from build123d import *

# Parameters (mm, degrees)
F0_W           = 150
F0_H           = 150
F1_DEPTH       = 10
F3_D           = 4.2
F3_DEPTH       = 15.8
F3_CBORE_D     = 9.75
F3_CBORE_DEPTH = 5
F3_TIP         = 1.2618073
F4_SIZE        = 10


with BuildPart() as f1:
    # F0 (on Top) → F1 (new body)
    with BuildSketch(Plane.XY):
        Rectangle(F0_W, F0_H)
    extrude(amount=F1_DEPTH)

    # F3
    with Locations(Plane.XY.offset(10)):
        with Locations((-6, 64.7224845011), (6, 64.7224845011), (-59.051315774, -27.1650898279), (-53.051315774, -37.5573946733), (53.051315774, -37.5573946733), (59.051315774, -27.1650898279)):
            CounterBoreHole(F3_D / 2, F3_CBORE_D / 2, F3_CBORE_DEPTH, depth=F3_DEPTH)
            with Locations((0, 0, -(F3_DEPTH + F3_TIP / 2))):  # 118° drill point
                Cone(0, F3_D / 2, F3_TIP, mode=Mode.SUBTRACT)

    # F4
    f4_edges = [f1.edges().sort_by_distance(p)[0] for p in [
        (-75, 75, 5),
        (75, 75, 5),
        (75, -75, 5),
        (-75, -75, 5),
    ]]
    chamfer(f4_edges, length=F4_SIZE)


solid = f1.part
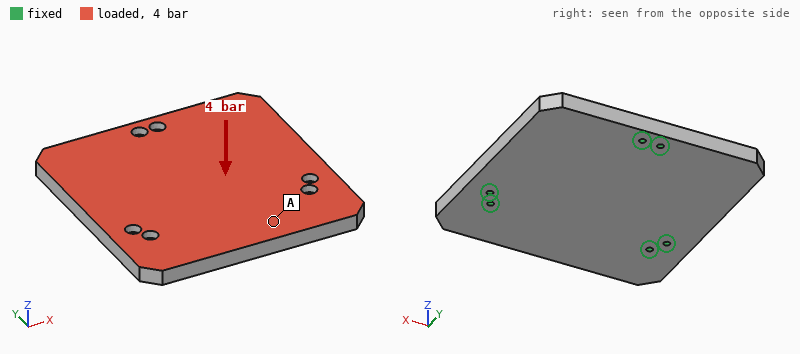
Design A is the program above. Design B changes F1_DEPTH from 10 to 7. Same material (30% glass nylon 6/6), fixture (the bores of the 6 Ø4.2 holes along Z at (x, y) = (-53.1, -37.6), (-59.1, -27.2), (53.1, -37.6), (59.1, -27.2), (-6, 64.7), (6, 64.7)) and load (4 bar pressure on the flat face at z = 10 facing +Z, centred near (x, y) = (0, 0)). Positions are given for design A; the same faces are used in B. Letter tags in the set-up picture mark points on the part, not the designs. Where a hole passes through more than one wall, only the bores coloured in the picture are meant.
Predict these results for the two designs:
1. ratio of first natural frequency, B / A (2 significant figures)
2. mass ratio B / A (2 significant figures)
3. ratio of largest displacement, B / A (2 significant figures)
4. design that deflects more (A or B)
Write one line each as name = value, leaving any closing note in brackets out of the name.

ratio of first natural frequency, B / A = 0.79
mass ratio B / A = 0.70
ratio of largest displacement, B / A = 2.6
design that deflects more = B
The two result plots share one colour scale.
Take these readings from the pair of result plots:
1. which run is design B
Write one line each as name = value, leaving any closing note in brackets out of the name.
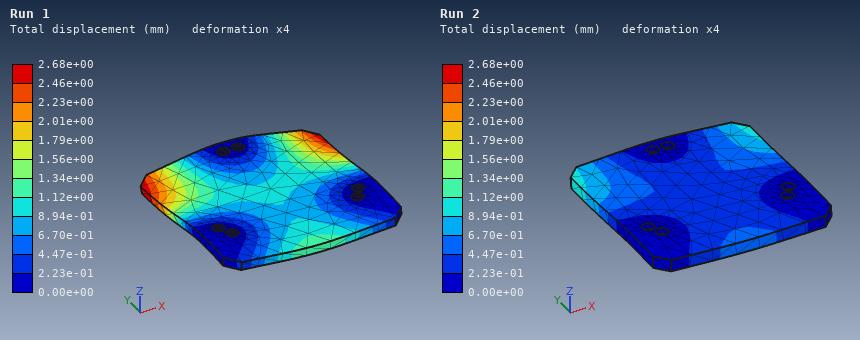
which run is design B = Run 1
